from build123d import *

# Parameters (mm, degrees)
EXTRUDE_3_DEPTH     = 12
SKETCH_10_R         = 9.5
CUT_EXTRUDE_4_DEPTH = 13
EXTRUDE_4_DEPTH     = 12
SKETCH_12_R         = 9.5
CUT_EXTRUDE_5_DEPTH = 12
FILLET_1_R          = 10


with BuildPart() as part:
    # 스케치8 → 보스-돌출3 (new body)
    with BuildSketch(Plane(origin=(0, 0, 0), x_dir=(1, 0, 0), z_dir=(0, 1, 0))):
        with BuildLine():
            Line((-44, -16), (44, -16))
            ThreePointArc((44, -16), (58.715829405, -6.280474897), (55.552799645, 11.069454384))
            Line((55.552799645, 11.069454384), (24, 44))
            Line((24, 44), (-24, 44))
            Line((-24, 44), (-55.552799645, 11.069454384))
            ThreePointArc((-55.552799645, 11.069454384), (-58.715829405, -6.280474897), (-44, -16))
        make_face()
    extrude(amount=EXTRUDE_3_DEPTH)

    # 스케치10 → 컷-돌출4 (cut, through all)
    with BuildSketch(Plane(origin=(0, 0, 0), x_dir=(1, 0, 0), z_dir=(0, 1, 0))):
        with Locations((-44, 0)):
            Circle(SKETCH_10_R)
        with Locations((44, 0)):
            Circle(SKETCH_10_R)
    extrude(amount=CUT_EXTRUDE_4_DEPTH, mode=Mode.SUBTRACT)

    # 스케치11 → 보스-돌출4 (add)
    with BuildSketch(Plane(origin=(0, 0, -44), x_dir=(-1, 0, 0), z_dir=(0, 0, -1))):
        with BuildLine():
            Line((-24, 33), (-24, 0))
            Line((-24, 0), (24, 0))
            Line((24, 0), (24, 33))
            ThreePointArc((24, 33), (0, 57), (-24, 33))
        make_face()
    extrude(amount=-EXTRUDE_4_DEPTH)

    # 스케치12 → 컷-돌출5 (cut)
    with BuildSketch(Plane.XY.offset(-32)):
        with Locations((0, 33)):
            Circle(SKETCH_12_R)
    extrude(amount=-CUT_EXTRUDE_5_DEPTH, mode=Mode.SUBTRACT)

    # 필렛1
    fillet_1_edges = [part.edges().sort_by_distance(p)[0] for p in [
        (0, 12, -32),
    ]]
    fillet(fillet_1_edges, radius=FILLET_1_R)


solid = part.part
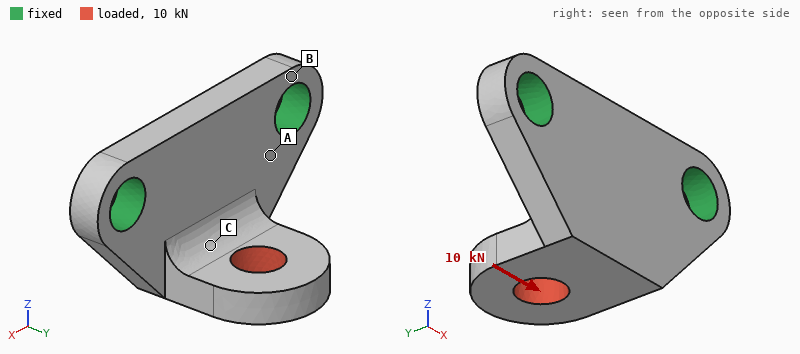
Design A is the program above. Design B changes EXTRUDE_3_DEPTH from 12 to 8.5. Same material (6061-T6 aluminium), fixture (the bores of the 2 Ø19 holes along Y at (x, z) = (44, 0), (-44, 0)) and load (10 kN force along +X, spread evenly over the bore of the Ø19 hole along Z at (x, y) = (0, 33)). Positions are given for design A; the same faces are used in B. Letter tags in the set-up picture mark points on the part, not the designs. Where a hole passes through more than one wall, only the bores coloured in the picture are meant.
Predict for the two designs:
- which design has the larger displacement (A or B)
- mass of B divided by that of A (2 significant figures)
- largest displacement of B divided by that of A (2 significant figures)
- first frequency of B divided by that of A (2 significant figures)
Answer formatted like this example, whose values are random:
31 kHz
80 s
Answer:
B
0.81
2.0
0.65
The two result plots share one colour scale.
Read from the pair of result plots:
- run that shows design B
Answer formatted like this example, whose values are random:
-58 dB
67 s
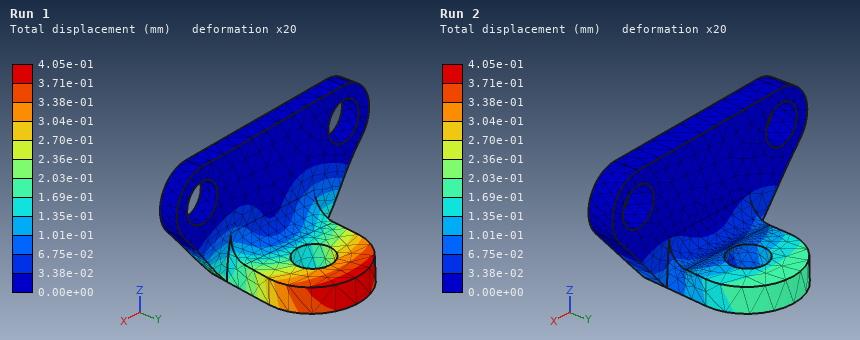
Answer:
Run 1
